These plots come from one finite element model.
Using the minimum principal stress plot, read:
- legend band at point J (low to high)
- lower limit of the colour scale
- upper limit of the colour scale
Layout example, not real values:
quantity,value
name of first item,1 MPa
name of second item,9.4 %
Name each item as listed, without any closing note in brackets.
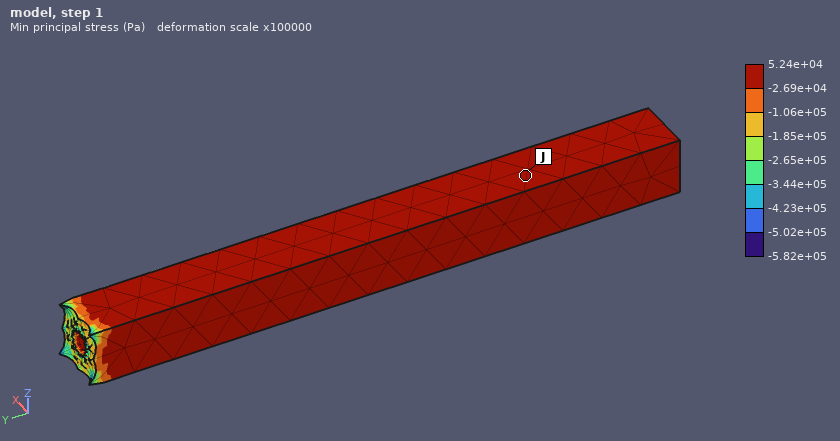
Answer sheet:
quantity,value
legend band at point J,-2.69e+04 to 5.24e+04 Pa
lower limit of the colour scale,-5.82e+05 Pa
upper limit of the colour scale,5.24e+04 Pa
